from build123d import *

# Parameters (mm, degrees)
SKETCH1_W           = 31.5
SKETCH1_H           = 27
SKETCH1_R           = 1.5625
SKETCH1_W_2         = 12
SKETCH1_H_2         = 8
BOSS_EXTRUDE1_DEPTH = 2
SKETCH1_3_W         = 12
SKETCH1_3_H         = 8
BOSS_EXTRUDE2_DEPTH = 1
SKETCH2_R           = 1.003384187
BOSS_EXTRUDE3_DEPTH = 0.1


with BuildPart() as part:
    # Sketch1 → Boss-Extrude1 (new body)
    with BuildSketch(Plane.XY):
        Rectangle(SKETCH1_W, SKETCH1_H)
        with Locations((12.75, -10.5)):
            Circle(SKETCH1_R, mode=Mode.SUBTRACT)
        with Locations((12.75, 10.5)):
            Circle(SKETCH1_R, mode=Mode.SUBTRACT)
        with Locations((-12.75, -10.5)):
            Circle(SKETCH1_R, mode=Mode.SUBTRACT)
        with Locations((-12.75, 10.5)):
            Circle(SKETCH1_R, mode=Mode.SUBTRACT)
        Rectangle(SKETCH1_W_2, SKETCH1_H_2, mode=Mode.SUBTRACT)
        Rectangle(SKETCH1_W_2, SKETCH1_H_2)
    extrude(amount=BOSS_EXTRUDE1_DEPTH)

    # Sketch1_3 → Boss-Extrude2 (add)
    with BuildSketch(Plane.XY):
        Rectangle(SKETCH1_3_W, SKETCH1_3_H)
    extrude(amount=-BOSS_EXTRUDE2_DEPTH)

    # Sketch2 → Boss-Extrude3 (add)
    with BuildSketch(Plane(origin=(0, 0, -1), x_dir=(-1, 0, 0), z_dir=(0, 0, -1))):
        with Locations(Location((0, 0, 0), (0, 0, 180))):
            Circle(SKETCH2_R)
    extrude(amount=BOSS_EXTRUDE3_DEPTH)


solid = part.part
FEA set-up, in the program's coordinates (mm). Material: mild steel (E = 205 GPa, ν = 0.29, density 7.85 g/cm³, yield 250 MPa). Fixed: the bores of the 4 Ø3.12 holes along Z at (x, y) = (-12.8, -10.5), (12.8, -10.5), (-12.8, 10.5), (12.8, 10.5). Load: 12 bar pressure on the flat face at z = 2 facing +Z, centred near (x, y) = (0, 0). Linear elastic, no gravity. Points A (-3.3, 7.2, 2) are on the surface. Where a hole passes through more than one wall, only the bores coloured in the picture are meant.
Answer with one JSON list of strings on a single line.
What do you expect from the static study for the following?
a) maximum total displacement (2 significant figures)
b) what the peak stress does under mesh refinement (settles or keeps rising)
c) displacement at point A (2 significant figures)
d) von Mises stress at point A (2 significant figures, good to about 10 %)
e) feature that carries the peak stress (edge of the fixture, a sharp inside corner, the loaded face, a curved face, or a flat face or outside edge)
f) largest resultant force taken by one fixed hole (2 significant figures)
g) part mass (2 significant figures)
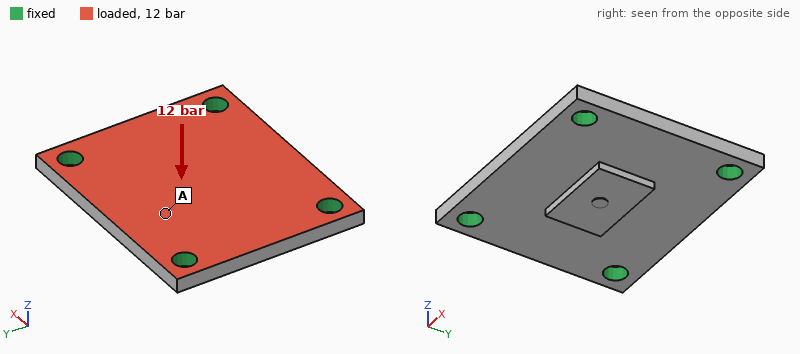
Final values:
["11 µm", "keeps rising", "9.2 µm", "35 MPa", "edge of the fixture", "250 N", "14 g"]
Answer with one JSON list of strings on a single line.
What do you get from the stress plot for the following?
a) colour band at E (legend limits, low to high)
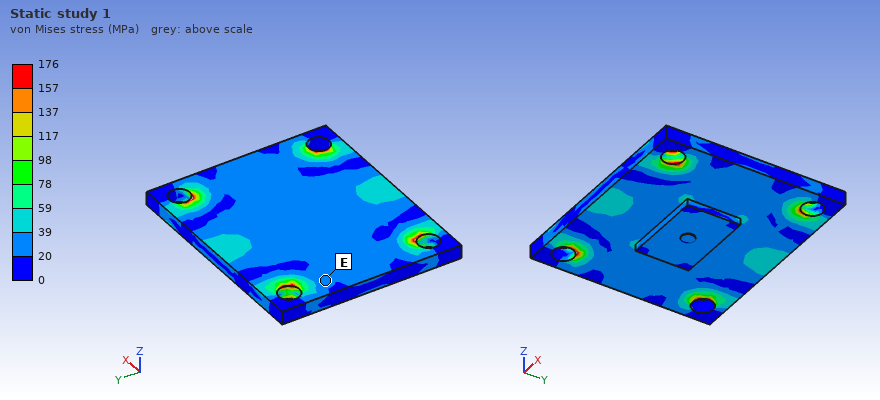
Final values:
["20 to 39 MPa"]
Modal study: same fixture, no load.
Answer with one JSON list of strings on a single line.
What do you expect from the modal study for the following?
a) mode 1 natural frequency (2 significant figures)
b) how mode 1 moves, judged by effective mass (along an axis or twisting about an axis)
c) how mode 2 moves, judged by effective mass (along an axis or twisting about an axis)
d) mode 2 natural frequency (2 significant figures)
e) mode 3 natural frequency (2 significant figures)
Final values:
["14 kHz", "along Z", "twisting about X", "21 kHz", "27 kHz"]
